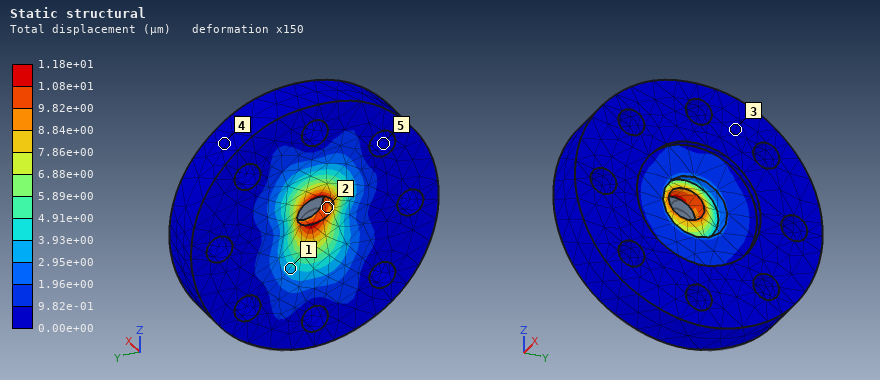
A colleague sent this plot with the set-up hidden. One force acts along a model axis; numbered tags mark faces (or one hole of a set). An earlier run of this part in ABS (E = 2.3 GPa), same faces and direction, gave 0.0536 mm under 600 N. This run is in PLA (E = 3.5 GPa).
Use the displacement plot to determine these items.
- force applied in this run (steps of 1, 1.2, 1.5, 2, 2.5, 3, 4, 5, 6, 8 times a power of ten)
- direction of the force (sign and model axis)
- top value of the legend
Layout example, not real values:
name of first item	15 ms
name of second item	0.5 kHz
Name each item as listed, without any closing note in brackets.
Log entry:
force applied in this run	200 N
direction of the force	+Z
top value of the legend	1.18e+01 µm
